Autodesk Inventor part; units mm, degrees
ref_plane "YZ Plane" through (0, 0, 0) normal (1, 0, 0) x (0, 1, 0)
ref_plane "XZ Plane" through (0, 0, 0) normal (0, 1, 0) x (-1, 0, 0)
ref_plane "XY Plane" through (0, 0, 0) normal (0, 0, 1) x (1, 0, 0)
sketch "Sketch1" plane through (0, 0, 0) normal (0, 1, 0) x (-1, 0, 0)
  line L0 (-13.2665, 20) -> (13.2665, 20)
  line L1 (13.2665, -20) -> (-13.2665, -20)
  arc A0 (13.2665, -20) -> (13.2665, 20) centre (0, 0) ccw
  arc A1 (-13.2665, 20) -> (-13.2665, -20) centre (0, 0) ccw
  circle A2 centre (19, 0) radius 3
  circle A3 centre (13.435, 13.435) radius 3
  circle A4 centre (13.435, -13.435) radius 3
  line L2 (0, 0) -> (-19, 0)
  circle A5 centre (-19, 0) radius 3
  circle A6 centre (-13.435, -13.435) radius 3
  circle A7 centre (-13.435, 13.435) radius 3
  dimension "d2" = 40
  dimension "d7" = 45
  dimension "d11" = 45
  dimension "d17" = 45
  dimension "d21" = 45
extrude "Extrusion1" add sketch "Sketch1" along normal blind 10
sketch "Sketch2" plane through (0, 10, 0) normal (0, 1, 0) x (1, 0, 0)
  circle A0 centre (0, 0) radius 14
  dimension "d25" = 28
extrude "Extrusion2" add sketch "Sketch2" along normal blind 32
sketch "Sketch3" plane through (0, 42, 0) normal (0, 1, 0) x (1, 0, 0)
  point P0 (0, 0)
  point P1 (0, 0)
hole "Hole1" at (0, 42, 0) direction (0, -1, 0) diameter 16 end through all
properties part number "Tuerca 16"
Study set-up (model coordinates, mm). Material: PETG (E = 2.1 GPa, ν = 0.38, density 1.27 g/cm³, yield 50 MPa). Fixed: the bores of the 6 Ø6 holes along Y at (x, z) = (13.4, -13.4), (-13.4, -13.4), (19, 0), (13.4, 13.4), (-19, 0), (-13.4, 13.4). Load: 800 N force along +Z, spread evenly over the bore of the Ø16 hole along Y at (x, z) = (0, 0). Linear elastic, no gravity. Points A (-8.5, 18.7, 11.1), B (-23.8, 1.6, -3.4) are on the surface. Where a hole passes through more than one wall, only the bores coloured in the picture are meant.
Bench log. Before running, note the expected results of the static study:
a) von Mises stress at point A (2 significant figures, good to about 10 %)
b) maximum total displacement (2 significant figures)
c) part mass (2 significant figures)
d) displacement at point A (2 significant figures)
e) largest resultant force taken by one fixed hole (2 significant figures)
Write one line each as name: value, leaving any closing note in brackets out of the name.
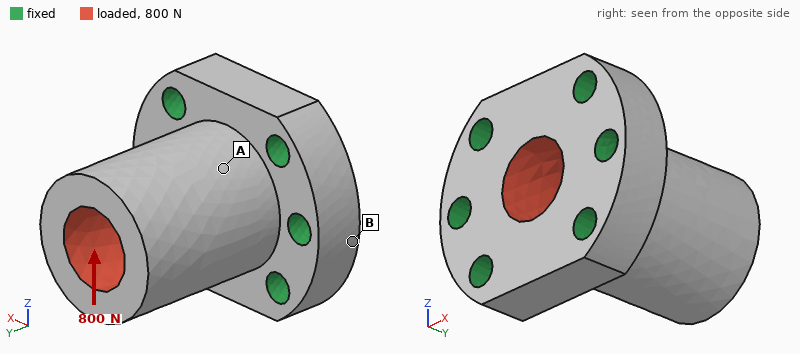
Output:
von Mises stress at point A: 2.4 MPa
maximum total displacement: 0.16 mm
part mass: 33 g
displacement at point A: 0.060 mm
largest resultant force taken by one fixed hole: 300 N
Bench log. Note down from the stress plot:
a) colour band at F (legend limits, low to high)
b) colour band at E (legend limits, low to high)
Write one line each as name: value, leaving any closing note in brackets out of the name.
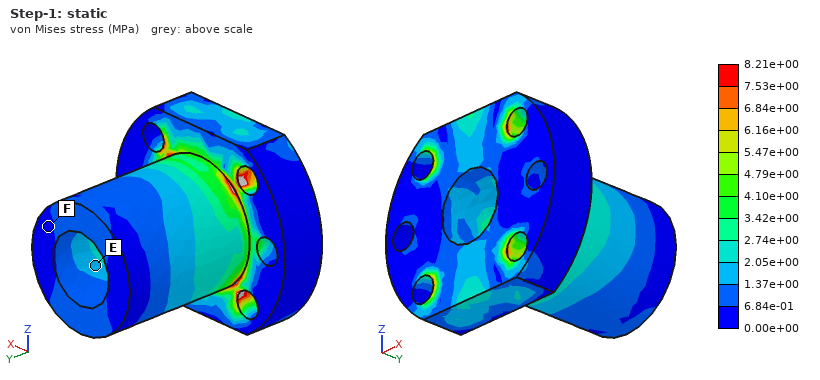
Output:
colour band at F: 0.00e+00 to 6.84e-01 MPa
colour band at E: 1.37e+00 to 2.05e+00 MPa
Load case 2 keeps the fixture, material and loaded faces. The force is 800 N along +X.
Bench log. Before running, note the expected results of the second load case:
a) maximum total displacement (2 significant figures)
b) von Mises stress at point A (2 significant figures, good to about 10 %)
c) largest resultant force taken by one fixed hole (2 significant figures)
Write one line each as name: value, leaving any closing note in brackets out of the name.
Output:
maximum total displacement: 0.14 mm
von Mises stress at point A: 2.4 MPa
largest resultant force taken by one fixed hole: 260 N
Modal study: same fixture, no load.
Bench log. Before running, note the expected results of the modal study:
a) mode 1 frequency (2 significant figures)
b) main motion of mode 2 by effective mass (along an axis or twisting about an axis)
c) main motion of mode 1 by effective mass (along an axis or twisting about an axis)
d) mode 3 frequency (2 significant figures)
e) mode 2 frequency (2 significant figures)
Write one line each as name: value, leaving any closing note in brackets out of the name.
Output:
mode 1 frequency: 2800 Hz
main motion of mode 2 by effective mass: along X
main motion of mode 1 by effective mass: along Z
mode 3 frequency: 5500 Hz
mode 2 frequency: 3100 Hz
